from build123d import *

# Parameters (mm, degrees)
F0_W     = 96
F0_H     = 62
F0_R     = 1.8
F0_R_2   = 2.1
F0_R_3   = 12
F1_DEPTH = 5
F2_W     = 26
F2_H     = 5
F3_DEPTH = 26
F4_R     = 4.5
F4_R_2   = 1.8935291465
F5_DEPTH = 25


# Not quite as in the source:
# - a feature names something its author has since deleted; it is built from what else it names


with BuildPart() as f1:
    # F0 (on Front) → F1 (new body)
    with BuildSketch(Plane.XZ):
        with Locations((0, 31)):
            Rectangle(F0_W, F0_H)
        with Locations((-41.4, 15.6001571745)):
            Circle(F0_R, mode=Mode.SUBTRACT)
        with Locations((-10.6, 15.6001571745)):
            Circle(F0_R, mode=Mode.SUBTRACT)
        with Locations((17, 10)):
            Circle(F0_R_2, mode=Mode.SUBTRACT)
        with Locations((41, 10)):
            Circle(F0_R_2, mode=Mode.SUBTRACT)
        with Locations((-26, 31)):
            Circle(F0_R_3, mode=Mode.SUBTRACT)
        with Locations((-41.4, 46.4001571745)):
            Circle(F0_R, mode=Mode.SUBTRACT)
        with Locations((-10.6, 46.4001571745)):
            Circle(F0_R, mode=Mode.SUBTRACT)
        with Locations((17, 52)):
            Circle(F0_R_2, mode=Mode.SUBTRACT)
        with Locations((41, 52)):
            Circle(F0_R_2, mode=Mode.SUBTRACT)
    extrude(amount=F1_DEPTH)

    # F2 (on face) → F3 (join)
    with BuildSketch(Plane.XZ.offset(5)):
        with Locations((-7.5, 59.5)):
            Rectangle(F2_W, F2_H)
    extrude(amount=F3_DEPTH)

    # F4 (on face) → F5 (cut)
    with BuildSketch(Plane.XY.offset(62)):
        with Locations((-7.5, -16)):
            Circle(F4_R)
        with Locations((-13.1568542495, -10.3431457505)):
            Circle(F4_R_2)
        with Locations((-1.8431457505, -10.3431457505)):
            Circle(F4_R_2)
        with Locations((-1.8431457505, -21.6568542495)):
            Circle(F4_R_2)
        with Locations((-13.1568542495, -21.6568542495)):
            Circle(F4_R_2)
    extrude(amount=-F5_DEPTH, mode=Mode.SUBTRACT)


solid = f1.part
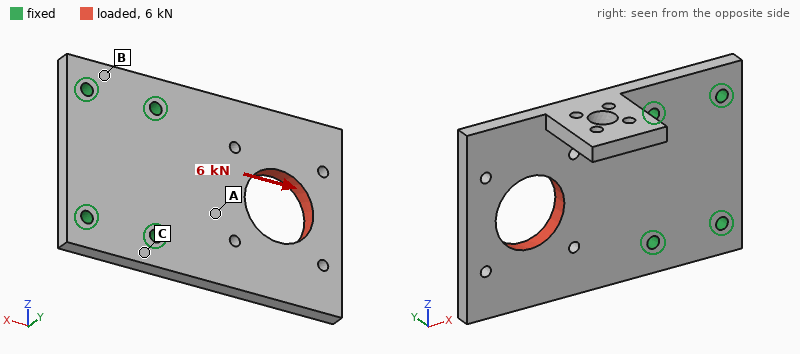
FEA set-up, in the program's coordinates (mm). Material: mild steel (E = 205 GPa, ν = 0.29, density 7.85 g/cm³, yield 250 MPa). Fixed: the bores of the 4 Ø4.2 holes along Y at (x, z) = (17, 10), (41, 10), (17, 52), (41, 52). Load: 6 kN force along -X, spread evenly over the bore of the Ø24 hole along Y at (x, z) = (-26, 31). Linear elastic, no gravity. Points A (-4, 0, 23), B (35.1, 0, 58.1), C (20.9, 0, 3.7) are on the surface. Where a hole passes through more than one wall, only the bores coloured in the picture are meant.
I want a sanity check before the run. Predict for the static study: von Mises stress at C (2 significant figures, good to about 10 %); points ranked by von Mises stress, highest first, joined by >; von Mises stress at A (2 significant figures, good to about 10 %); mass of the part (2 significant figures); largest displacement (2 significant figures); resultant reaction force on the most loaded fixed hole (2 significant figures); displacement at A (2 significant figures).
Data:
12 MPa
A > C > B
22 MPa
230 g
11 µm
2.4 kN
2.8 µm
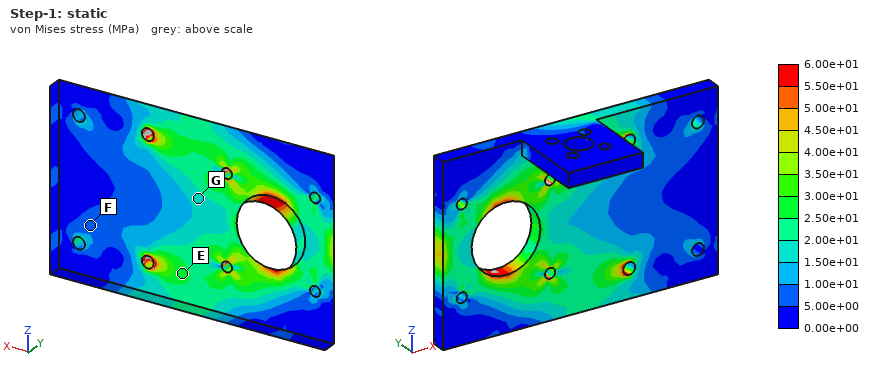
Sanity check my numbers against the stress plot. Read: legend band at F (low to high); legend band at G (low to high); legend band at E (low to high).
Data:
5.00e+00 to 1.00e+01 MPa
1.50e+01 to 2.00e+01 MPa
2.50e+01 to 3.00e+01 MPa
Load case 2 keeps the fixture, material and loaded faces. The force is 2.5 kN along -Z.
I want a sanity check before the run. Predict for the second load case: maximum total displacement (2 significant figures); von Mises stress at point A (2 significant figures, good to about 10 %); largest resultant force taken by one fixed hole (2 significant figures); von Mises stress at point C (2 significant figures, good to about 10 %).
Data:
19 µm
22 MPa
2.4 kN
18 MPa
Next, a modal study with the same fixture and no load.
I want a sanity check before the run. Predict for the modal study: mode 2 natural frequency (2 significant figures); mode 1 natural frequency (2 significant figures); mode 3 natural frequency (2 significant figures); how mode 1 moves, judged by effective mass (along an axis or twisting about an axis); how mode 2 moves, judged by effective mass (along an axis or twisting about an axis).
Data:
2000 Hz
1000 Hz
3400 Hz
along Y
twisting about X
